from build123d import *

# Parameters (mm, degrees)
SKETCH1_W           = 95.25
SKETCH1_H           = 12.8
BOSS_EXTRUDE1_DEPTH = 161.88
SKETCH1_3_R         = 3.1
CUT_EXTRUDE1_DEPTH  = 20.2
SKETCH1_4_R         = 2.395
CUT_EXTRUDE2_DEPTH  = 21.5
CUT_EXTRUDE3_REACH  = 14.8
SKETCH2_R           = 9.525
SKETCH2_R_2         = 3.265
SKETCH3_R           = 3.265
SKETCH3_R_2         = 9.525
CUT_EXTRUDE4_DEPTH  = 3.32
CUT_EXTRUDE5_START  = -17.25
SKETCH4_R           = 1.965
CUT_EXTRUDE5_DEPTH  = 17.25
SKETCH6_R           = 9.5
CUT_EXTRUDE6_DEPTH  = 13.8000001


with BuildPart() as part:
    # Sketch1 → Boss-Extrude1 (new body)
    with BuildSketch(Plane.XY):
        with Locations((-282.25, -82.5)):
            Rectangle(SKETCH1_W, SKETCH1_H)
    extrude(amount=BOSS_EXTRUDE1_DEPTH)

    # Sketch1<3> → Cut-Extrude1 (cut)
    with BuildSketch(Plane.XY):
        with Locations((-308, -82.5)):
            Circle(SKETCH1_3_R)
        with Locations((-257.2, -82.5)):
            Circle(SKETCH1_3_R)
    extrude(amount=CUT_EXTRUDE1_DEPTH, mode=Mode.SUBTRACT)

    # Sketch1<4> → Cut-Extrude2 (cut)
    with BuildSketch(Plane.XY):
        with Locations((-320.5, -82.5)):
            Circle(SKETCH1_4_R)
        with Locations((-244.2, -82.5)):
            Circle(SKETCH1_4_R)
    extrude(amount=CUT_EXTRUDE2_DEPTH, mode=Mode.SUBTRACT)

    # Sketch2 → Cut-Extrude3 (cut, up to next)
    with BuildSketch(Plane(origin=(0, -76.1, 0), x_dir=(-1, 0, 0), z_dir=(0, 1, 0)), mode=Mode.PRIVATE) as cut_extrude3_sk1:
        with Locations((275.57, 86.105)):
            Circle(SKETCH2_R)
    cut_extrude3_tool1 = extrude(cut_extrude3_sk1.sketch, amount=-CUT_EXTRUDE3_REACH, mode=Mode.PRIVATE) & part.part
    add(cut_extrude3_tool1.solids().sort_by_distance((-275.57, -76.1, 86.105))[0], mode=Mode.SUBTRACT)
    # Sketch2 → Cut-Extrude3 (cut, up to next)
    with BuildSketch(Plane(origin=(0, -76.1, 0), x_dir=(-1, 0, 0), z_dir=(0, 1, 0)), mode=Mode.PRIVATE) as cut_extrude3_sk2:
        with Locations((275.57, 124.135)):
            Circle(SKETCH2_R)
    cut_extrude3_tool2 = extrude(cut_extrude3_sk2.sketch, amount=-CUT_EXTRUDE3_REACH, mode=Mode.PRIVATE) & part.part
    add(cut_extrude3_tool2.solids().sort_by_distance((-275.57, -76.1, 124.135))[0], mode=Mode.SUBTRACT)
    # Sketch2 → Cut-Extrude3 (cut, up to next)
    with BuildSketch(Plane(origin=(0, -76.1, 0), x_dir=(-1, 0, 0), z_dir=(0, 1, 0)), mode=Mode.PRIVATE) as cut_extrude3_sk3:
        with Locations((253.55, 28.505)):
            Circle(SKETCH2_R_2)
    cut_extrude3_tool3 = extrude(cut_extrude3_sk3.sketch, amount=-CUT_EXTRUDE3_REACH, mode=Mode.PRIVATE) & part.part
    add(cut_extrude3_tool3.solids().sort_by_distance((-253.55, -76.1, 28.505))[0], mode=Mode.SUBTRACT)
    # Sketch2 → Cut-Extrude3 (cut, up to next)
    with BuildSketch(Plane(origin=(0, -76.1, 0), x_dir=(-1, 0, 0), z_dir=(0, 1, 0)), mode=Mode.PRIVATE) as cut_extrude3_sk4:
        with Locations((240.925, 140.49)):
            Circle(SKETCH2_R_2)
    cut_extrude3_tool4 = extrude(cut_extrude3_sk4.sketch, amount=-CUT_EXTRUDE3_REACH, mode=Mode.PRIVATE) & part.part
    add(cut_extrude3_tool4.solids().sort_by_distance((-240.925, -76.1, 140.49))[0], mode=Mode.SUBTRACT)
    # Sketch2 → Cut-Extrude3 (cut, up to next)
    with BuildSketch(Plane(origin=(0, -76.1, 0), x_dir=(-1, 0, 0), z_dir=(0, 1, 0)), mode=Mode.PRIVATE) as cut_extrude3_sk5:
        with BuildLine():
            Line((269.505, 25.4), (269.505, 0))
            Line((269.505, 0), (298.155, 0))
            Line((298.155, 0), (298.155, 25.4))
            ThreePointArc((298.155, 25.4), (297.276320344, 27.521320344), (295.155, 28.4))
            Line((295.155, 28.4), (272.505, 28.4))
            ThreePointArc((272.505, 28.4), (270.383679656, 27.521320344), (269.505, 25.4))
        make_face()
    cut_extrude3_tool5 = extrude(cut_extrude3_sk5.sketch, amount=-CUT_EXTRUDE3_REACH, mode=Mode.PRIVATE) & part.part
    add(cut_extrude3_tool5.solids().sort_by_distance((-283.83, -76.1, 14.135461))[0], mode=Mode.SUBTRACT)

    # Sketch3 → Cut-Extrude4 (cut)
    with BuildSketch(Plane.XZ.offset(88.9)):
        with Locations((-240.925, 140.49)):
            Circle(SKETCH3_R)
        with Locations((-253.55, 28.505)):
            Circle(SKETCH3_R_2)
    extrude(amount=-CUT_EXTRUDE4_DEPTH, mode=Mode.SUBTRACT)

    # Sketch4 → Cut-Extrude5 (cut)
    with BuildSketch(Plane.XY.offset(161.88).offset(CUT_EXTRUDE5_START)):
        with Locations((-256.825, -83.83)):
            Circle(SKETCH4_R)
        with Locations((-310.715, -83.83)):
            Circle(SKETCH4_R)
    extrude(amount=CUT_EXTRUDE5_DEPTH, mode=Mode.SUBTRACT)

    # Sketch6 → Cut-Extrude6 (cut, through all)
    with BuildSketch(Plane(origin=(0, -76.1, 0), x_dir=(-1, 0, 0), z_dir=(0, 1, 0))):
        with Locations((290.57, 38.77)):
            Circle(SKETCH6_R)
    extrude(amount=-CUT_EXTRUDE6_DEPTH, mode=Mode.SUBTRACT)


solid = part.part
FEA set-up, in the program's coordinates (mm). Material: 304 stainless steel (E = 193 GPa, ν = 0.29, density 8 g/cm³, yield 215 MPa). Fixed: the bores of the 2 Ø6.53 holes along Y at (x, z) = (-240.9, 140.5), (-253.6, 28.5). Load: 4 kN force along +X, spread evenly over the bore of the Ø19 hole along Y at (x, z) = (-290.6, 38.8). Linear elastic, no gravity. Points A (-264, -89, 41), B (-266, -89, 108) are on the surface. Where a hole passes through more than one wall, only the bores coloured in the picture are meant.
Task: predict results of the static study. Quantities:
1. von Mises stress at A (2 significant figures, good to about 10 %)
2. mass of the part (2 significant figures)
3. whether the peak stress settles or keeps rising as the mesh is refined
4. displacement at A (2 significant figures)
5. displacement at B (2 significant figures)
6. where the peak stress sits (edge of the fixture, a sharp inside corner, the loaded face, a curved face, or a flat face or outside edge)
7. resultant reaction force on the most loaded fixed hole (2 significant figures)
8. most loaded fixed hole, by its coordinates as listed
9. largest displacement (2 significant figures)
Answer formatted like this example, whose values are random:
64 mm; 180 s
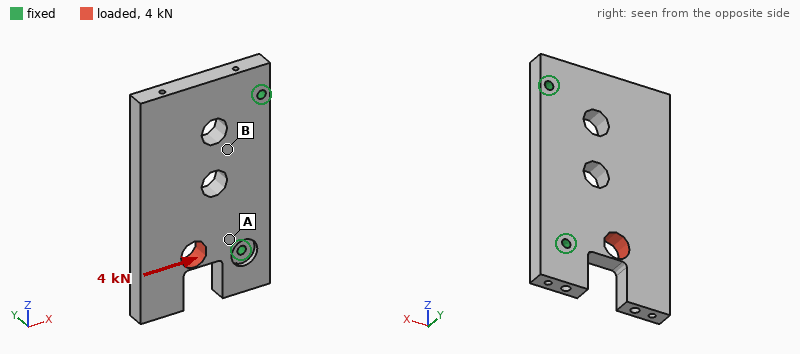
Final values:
8.0 MPa; 1.4 kg; keeps rising; 2.7 µm; 1.6 µm; a sharp inside corner; 3.6 kN; (-253.6, 28.5); 11 µm
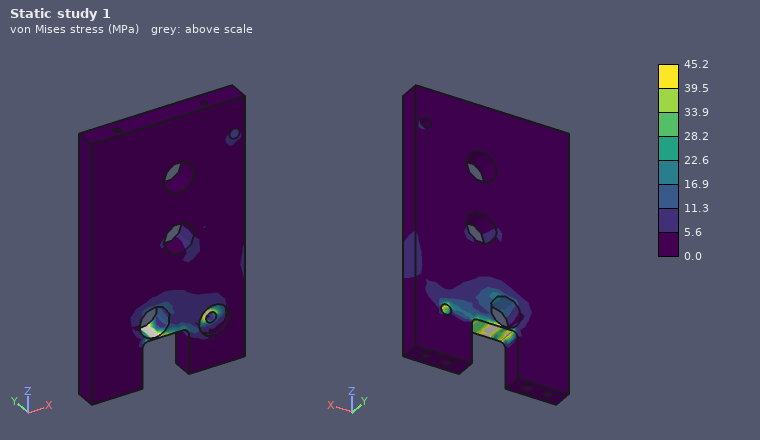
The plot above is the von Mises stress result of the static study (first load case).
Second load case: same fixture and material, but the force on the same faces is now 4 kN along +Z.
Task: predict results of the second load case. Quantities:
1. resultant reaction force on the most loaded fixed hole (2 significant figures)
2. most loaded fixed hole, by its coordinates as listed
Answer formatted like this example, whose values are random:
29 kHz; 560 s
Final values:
3.0 kN; (-253.6, 28.5)
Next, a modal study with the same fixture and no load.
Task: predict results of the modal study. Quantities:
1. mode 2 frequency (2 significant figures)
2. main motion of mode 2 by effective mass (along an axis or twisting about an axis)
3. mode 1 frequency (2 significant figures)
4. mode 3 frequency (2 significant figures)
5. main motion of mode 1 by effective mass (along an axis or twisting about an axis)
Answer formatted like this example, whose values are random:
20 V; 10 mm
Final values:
1700 Hz; twisting about X; 880 Hz; 3100 Hz; along Y
